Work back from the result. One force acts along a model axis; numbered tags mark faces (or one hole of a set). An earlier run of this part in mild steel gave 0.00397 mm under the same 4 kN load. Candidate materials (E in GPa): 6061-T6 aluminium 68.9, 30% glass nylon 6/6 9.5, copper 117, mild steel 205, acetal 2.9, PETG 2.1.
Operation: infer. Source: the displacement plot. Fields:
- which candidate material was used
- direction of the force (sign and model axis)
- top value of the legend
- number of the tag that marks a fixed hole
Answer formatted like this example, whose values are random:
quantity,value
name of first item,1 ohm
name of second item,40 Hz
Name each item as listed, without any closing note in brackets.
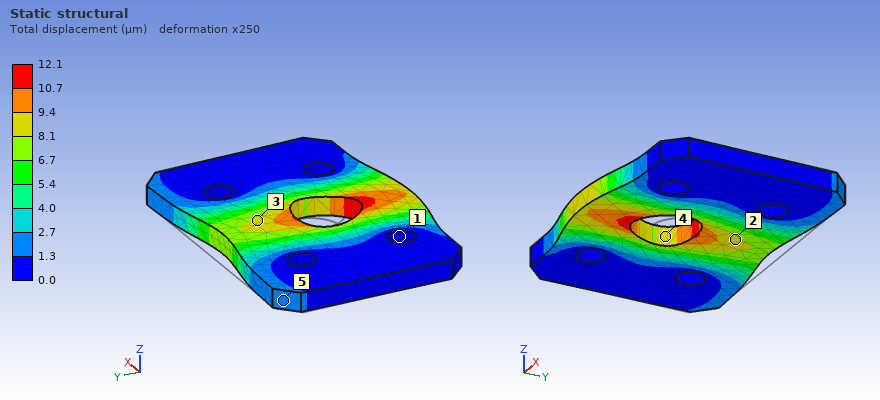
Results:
quantity,value
which candidate material was used,6061-T6 aluminium
direction of the force,-Y
top value of the legend,12.1 µm
number of the tag that marks a fixed hole,1
